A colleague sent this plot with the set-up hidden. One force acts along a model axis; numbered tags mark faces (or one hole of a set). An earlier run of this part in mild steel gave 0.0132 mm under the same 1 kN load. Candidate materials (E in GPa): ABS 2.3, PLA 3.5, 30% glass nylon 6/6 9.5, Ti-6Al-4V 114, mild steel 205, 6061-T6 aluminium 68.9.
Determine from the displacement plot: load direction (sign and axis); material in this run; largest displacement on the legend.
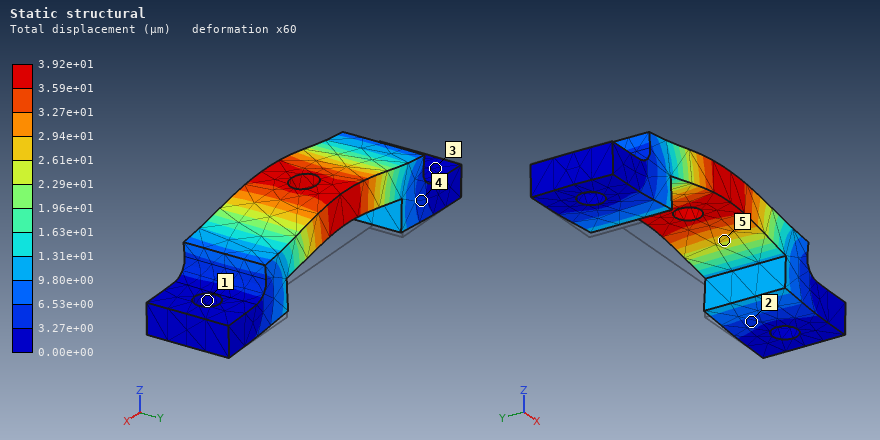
+Z
6061-T6 aluminium
3.92e+01 µm
